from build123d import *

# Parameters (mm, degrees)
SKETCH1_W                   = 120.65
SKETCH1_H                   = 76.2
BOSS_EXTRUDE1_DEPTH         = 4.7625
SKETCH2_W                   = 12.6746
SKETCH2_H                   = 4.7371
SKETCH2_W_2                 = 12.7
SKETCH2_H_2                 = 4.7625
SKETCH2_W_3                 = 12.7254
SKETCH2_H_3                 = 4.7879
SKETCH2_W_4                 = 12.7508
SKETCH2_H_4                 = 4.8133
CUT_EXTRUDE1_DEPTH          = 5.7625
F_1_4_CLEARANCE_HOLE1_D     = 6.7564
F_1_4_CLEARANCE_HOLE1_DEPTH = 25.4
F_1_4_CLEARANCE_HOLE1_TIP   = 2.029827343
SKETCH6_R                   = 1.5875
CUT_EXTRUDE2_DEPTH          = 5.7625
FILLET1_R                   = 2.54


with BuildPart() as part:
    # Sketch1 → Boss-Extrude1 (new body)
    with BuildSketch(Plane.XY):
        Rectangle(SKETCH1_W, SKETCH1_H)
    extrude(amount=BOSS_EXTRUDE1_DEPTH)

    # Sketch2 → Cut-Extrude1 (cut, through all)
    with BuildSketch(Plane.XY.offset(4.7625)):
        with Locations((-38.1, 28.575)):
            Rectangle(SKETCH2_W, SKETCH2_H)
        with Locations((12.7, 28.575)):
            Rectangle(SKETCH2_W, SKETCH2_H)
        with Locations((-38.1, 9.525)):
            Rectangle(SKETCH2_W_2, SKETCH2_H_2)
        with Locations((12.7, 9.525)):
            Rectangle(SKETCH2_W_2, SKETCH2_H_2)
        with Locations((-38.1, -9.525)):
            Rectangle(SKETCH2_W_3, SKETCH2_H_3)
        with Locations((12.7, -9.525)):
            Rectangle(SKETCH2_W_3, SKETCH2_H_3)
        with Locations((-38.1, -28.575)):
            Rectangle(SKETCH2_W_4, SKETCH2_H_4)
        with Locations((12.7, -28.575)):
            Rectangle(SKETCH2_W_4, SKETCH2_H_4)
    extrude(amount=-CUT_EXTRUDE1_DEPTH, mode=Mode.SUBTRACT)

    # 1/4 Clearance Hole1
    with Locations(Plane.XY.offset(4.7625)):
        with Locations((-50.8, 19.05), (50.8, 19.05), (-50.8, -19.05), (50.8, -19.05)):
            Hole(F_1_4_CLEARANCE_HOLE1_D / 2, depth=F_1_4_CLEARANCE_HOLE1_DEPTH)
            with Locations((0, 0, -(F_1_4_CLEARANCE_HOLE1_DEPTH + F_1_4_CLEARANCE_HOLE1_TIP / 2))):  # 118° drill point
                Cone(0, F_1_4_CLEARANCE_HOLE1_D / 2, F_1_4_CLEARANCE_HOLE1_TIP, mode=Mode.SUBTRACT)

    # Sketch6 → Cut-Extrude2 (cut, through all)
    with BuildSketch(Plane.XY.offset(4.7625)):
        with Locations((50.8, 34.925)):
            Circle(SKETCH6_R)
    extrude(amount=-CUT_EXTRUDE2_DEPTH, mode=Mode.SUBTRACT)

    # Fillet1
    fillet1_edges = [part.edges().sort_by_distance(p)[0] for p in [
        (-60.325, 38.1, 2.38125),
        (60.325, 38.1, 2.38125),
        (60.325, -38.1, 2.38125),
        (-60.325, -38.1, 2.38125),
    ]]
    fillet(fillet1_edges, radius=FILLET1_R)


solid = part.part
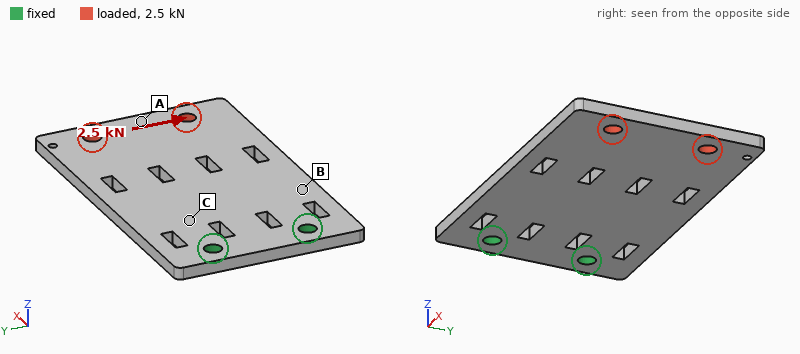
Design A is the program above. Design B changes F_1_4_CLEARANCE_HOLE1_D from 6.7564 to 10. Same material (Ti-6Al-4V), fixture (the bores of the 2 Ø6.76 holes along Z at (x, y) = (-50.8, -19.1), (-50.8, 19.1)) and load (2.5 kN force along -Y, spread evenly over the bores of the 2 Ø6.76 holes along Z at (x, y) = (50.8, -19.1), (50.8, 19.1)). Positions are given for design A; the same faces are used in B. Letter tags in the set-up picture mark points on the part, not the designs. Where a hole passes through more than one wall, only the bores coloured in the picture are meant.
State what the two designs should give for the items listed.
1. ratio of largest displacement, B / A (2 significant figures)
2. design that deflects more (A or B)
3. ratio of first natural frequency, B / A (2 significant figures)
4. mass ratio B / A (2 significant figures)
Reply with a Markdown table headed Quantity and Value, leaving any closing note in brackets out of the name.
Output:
| Quantity | Value |
|---|---|
| ratio of largest displacement, B / A | 0.88 |
| design that deflects more | A |
| ratio of first natural frequency, B / A | 1.1 |
| mass ratio B / A | 0.98 |
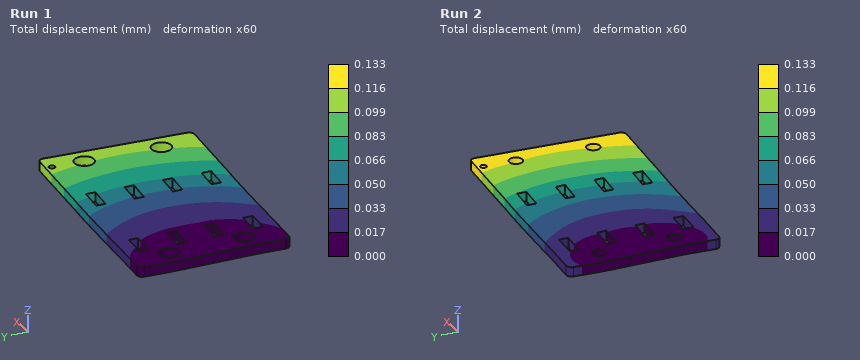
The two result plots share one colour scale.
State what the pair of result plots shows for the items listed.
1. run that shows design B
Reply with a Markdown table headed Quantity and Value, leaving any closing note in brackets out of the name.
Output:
| Quantity | Value |
|---|---|
| run that shows design B | Run 1 |
